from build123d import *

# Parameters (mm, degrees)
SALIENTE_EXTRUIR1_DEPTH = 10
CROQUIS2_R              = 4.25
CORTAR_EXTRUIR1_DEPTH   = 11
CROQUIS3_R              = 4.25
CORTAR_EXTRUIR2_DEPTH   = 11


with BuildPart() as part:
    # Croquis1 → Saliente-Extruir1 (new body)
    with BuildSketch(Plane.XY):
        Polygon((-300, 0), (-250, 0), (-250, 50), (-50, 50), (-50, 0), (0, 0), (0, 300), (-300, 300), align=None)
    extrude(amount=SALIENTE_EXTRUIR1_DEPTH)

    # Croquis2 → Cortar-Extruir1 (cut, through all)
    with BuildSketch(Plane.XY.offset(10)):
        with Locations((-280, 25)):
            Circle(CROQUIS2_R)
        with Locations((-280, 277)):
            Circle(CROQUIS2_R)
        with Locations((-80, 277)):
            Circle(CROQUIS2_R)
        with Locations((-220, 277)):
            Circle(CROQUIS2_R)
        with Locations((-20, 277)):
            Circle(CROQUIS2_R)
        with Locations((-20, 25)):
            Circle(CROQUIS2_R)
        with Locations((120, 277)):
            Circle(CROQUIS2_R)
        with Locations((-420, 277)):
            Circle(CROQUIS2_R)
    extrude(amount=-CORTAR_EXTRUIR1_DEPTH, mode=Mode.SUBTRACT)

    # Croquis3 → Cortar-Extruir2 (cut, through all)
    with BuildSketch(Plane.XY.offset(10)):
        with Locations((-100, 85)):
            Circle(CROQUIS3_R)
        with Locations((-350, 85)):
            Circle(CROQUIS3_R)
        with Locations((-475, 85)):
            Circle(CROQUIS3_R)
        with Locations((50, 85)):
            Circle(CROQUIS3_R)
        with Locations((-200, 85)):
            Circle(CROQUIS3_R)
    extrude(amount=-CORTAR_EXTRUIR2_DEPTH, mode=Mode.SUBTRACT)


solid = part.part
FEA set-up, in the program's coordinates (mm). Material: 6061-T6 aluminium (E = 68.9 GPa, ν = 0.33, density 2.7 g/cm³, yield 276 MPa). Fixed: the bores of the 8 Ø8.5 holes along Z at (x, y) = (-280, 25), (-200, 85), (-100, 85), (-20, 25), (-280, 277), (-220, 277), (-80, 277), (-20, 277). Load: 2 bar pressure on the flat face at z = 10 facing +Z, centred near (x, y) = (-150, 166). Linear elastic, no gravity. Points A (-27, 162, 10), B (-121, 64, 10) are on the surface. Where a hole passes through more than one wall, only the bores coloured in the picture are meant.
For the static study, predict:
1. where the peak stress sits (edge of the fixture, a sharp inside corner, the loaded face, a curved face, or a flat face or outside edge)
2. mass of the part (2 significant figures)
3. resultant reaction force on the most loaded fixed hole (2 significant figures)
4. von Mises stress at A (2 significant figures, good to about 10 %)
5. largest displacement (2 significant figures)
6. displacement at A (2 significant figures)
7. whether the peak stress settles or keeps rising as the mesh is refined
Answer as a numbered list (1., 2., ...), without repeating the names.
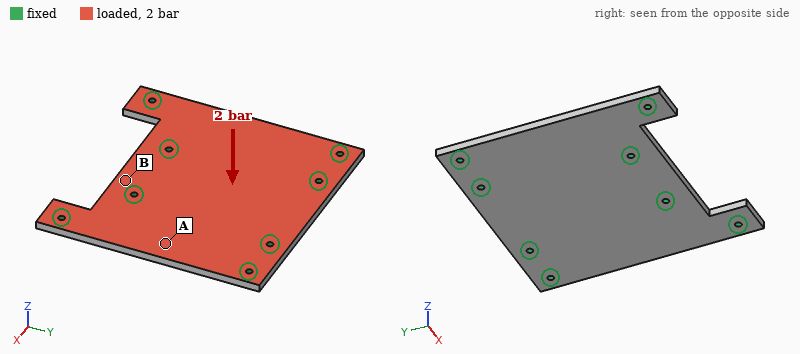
1. edge of the fixture
2. 2.1 kg
3. 3.2 kN
4. 23 MPa
5. 0.30 mm
6. 0.25 mm
7. keeps rising
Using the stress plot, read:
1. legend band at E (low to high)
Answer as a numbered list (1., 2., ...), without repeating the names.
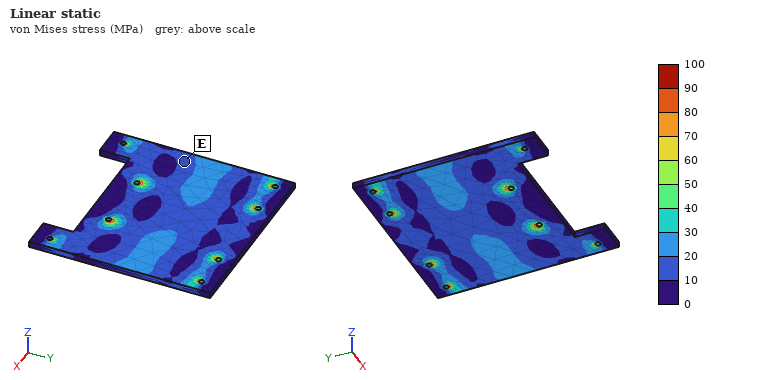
1. 10 to 20 MPa
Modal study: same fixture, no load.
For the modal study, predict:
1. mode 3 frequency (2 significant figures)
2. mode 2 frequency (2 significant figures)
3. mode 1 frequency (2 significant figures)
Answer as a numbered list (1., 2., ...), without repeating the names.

1. 1400 Hz
2. 1100 Hz
3. 1000 Hz
